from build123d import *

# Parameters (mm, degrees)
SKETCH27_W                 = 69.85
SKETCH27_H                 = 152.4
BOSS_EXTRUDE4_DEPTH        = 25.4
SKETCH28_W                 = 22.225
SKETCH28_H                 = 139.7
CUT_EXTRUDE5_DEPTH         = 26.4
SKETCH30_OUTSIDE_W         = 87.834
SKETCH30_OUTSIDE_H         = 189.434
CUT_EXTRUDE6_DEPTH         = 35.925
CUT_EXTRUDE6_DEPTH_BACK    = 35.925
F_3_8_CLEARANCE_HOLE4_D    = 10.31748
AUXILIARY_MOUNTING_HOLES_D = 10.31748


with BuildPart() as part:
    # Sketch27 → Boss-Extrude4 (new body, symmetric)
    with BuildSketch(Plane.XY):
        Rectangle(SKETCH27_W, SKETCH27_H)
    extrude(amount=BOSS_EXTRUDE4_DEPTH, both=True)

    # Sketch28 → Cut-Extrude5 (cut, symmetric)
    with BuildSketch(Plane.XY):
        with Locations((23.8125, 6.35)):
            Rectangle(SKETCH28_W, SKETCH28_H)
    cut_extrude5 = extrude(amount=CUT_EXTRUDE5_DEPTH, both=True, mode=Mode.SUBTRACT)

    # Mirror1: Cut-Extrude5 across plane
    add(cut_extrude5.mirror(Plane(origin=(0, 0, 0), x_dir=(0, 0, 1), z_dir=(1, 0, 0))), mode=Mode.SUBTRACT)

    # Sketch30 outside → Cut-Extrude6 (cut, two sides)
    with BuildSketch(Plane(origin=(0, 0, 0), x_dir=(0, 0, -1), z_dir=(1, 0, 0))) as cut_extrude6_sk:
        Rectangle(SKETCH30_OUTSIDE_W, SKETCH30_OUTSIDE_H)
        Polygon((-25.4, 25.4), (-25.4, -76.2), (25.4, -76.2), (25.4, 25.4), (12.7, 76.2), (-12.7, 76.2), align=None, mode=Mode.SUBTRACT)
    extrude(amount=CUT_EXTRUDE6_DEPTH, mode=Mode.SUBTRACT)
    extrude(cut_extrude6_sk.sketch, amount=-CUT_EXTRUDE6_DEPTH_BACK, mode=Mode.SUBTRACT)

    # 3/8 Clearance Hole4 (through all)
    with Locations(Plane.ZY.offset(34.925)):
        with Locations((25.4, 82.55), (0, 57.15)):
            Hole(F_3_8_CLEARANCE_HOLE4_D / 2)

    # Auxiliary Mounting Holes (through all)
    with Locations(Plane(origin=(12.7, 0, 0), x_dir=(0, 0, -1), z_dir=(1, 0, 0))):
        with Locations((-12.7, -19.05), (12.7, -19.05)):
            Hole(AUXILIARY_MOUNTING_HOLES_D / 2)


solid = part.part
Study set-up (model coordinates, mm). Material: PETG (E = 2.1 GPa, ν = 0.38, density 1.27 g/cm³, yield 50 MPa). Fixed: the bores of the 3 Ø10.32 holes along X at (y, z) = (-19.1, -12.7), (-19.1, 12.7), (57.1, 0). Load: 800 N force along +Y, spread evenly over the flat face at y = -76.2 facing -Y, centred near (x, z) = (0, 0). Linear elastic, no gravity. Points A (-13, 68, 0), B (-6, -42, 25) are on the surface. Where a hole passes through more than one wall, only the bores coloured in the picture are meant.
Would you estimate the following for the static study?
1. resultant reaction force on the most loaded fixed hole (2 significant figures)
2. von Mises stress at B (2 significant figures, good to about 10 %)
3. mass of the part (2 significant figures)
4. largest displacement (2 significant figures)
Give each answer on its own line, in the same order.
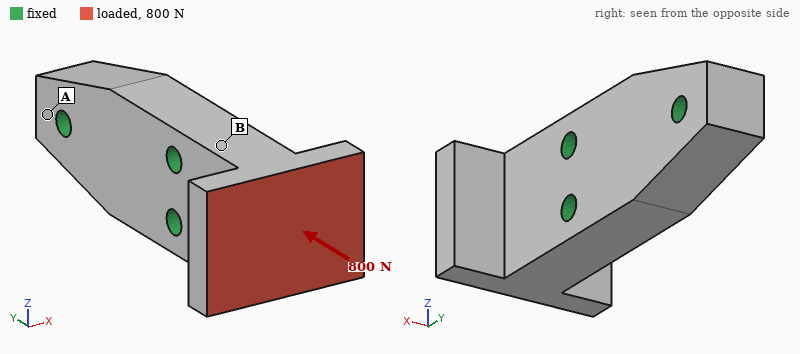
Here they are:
400 N
0.49 MPa
260 g
68 µm
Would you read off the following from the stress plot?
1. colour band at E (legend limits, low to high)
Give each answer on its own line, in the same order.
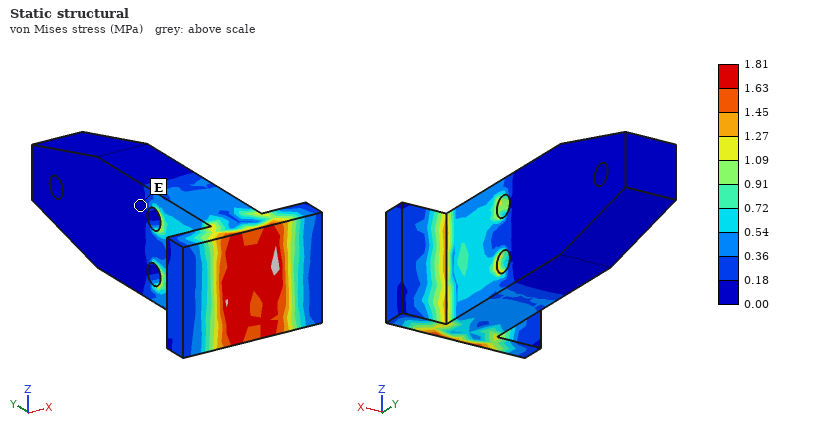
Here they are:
0.00 to 0.18 MPa
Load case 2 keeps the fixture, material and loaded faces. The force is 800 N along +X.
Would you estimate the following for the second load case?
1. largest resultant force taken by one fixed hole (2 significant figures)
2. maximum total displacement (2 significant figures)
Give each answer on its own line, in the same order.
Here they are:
420 N
0.48 mm
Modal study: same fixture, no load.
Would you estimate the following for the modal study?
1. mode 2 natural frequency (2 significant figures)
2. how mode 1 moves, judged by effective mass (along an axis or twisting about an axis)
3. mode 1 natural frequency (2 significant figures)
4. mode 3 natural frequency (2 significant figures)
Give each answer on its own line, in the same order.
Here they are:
1500 Hz
along X
950 Hz
1500 Hz
